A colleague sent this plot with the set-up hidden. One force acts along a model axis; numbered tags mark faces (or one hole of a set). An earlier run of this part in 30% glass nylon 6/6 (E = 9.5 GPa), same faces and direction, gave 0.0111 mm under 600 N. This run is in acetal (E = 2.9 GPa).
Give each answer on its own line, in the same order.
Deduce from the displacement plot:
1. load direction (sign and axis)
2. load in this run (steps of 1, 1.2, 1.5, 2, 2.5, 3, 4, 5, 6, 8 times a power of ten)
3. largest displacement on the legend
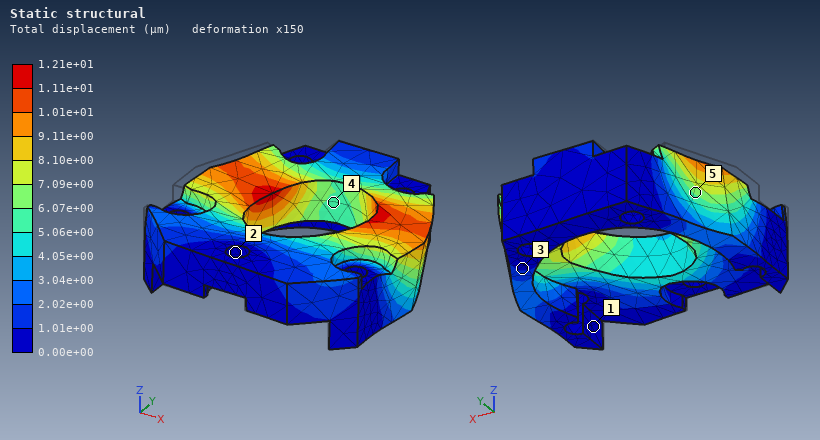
+X
200 N
1.21e+01 µm
